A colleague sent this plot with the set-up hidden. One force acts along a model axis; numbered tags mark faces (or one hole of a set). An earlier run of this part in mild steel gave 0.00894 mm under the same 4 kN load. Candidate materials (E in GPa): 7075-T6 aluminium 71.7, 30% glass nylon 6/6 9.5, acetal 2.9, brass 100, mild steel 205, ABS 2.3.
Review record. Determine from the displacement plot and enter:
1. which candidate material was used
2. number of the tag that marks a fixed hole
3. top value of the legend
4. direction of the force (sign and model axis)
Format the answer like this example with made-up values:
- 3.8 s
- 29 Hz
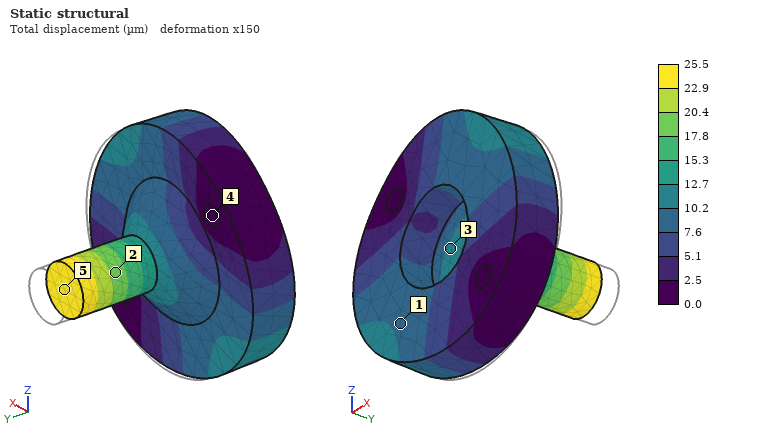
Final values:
- 7075-T6 aluminium
- 4
- 25.5 µm
- -Y
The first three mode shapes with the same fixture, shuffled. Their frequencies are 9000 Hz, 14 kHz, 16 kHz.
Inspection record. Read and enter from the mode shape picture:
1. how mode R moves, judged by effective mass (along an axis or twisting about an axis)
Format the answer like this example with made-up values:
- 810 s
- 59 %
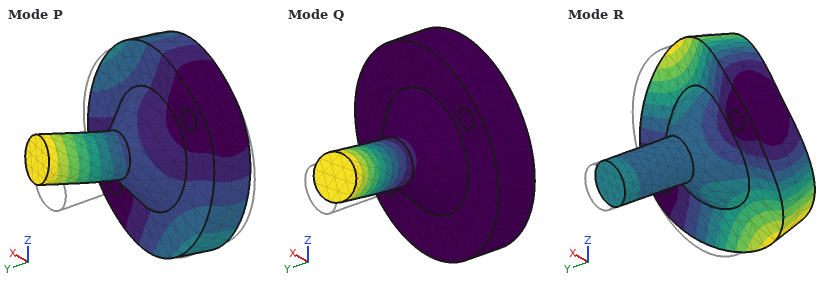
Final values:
- along Y
